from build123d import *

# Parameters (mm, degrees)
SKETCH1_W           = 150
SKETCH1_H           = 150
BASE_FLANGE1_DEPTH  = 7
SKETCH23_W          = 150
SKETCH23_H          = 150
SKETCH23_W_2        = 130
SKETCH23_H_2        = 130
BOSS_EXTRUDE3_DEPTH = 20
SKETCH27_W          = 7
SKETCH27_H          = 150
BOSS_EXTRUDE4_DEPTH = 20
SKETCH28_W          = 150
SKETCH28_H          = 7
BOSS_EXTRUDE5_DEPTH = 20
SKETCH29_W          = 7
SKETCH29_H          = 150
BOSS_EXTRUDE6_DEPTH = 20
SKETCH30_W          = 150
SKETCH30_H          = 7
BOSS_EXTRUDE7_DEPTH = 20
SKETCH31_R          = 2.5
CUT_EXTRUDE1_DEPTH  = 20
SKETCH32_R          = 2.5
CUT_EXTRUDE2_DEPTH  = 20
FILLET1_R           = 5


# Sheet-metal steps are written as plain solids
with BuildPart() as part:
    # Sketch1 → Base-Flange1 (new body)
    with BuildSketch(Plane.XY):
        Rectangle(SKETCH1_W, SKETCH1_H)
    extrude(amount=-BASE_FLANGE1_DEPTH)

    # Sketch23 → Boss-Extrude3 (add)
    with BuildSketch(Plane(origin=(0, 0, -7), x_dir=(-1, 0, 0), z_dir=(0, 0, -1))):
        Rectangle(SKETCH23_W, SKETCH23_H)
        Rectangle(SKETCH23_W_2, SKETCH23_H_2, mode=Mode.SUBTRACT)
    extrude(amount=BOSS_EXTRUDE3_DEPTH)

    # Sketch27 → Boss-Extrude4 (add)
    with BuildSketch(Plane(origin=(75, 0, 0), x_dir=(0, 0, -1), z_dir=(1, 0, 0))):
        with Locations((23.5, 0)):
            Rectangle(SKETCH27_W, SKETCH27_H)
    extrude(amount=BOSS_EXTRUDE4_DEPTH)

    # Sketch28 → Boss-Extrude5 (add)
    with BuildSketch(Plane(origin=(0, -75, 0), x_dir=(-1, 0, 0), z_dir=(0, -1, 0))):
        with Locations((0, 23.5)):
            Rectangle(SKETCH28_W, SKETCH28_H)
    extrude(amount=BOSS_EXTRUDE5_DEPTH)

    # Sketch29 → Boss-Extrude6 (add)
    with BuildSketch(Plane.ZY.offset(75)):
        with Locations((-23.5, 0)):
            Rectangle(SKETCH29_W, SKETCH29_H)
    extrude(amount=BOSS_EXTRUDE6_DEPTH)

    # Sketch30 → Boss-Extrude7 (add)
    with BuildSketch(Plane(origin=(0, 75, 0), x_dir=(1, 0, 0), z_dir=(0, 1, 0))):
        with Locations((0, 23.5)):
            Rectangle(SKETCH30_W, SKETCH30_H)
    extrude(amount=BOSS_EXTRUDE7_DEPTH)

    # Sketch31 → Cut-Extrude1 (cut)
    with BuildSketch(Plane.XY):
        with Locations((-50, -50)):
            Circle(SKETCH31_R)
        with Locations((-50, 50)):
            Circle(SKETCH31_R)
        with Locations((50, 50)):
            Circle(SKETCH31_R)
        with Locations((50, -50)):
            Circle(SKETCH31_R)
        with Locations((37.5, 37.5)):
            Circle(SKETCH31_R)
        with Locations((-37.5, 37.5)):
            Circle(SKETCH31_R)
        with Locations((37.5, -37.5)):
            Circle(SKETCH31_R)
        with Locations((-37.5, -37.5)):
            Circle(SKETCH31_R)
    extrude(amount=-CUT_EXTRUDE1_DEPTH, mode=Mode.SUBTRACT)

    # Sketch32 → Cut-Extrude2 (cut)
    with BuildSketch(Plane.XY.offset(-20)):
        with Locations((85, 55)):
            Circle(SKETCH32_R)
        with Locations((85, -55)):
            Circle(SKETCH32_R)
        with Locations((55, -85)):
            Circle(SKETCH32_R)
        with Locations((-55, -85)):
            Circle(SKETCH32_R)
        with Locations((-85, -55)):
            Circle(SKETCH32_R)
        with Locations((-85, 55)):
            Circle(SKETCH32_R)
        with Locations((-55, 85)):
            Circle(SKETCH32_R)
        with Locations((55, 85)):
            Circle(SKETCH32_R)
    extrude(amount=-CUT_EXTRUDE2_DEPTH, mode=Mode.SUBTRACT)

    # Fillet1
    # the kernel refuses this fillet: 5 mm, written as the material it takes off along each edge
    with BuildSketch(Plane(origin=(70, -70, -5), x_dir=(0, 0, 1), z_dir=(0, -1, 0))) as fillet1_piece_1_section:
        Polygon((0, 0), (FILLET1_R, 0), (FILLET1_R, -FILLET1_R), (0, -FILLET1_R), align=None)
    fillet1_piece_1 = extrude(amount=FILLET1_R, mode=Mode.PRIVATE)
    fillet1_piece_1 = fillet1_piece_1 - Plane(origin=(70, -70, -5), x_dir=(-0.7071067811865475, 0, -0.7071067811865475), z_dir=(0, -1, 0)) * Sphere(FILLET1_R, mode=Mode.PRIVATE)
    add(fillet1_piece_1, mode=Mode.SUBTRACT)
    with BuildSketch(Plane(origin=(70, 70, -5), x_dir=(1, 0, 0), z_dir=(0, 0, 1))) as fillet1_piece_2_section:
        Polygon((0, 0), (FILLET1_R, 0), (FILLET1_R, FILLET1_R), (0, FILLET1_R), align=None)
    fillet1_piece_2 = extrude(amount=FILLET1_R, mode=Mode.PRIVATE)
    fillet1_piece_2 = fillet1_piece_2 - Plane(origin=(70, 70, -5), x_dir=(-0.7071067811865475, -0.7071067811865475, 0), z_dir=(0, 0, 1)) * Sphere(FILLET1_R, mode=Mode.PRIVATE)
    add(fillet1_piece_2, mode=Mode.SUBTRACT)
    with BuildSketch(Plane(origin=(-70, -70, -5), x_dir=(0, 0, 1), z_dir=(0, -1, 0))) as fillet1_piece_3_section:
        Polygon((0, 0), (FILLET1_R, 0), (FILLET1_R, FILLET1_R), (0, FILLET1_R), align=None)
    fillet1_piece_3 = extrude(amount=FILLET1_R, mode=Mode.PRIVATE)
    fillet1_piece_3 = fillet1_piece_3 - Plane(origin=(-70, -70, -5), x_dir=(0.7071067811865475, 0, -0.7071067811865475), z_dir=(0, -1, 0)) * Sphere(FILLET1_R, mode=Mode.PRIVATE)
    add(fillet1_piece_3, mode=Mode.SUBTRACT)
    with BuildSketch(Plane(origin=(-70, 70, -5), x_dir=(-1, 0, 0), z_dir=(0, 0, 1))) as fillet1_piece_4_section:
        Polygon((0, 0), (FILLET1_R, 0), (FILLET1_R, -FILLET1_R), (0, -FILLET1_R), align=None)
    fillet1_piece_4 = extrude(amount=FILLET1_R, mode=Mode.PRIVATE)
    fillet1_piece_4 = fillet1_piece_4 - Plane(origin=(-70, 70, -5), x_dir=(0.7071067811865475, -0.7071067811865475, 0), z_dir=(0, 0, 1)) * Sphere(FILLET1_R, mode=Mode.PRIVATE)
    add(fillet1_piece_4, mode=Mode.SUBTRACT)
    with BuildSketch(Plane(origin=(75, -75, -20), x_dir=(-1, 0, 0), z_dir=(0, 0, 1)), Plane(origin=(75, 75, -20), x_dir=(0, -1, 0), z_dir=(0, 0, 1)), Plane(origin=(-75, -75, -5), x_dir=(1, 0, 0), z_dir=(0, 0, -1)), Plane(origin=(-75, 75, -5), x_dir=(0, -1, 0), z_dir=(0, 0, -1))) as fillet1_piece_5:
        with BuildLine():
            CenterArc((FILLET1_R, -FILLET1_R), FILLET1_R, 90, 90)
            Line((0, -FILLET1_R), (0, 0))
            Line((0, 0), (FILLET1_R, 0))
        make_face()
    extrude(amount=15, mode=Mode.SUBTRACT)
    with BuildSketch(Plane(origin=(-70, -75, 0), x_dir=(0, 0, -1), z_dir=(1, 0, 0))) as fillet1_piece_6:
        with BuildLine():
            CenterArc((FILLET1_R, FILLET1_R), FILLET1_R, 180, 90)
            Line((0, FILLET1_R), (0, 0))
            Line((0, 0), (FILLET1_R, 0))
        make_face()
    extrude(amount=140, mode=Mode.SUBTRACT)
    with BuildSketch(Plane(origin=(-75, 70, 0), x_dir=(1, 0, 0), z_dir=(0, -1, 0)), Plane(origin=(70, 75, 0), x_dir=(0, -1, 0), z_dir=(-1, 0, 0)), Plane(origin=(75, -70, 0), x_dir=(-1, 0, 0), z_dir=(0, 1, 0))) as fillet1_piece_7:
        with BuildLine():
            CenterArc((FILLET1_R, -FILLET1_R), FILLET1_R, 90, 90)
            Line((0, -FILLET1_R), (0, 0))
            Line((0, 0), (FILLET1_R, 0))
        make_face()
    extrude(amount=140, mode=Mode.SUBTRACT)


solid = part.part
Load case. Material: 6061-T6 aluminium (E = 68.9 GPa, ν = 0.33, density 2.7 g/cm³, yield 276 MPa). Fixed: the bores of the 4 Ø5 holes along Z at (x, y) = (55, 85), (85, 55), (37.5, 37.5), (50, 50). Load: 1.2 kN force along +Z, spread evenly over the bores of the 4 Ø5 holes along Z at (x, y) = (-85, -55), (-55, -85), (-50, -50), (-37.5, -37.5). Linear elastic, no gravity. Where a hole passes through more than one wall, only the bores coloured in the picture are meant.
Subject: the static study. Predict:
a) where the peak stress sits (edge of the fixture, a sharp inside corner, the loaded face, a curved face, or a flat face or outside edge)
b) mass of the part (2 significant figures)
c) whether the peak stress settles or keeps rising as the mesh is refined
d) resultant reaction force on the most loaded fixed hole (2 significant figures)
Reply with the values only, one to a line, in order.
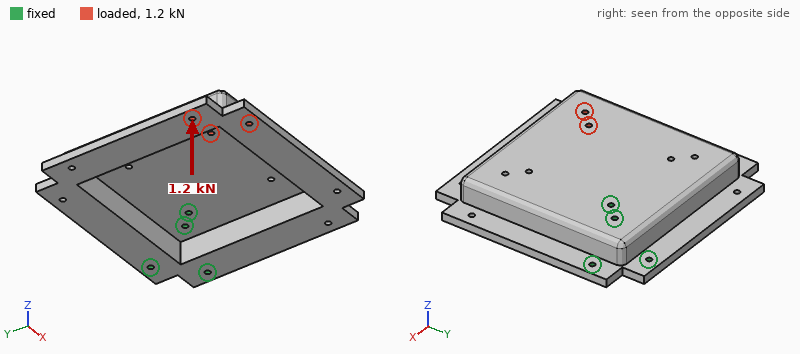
edge of the fixture
940 g
keeps rising
3.5 kN
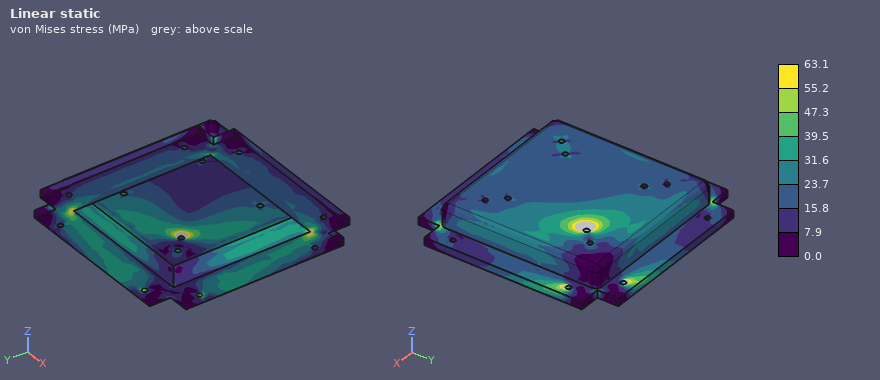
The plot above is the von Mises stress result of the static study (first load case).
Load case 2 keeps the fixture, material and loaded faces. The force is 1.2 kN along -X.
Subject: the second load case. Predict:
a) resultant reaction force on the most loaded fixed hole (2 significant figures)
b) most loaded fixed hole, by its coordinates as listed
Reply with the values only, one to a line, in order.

3.1 kN
(37.5, 37.5)
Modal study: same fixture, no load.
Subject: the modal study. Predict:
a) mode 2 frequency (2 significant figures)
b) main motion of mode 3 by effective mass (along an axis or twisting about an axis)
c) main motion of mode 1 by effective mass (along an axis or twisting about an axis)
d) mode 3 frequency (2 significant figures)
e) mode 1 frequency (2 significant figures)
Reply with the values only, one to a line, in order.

540 Hz
along Z
along Z
1100 Hz
360 Hz
